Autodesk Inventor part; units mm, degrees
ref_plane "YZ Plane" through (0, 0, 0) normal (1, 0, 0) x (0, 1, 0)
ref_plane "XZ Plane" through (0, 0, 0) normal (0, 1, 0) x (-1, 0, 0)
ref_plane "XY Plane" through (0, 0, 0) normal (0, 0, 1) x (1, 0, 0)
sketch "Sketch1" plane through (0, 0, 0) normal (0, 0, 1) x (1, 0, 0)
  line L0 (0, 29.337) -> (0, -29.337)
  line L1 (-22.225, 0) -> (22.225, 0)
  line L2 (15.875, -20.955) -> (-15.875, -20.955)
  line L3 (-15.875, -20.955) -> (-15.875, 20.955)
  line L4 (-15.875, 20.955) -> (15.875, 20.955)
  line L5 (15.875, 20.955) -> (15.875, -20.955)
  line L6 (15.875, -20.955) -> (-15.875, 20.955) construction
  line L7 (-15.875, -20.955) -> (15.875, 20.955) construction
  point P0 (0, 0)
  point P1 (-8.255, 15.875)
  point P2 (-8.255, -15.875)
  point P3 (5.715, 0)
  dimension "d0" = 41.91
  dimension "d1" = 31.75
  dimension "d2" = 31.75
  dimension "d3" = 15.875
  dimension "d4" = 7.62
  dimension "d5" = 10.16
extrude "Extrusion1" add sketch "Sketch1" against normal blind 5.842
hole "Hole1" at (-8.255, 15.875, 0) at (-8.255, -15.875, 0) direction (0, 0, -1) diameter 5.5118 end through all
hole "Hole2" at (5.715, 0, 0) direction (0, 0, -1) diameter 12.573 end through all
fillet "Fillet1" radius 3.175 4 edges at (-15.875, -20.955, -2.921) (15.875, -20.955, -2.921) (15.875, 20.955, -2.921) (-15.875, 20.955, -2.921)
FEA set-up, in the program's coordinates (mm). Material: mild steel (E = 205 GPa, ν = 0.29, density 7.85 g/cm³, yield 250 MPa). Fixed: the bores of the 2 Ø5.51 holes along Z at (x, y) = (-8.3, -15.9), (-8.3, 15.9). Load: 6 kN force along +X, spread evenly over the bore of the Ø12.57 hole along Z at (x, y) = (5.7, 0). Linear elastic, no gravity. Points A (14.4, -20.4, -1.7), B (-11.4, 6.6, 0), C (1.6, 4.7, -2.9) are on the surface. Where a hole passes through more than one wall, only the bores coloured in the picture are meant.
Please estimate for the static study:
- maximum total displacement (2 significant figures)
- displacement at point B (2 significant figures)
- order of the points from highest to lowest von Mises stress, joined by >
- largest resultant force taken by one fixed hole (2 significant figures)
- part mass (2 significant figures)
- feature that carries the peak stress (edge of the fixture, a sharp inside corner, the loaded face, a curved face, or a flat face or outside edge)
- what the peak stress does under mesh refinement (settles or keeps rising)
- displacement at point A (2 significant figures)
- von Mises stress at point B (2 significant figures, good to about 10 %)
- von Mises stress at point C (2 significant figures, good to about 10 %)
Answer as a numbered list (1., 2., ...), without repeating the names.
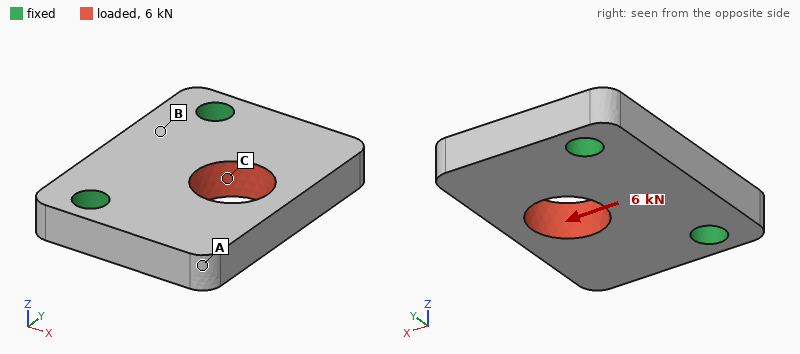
1. 7.7 µm
2. 2.2 µm
3. C > B > A
4. 3.2 kN
5. 53 g
6. edge of the fixture
7. keeps rising
8. 1.8 µm
9. 19 MPa
10. 38 MPa
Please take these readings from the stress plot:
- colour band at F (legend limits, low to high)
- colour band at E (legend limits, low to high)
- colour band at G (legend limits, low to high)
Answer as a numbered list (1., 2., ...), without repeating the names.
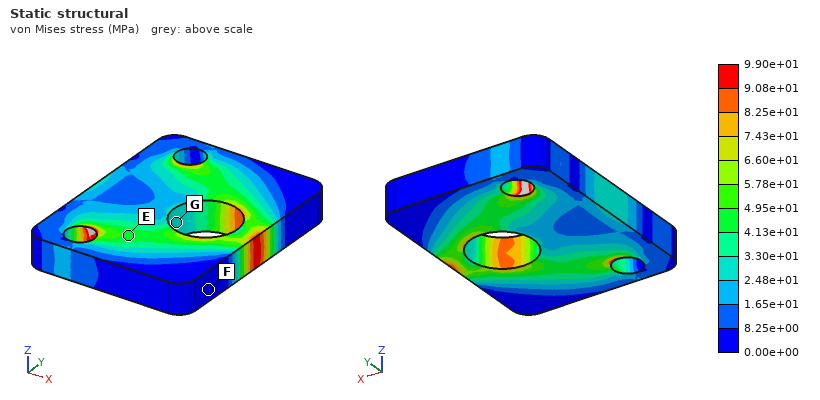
1. 0.00e+00 to 8.25e+00 MPa
2. 4.13e+01 to 4.95e+01 MPa
3. 2.48e+01 to 3.30e+01 MPa
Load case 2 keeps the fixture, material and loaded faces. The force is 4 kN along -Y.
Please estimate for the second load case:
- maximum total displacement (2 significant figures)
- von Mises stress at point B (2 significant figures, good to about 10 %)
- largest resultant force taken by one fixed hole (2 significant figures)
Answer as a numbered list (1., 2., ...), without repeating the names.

1. 8.3 µm
2. 13 MPa
3. 2.5 kN
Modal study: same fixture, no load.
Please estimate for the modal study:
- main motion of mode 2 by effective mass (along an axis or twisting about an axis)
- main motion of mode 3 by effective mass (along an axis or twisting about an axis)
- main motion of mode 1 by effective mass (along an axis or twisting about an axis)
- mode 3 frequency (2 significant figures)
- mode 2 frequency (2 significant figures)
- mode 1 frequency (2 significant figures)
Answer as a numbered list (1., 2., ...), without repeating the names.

1. twisting about X
2. along Y
3. along Z
4. 22 kHz
5. 13 kHz
6. 7900 Hz
